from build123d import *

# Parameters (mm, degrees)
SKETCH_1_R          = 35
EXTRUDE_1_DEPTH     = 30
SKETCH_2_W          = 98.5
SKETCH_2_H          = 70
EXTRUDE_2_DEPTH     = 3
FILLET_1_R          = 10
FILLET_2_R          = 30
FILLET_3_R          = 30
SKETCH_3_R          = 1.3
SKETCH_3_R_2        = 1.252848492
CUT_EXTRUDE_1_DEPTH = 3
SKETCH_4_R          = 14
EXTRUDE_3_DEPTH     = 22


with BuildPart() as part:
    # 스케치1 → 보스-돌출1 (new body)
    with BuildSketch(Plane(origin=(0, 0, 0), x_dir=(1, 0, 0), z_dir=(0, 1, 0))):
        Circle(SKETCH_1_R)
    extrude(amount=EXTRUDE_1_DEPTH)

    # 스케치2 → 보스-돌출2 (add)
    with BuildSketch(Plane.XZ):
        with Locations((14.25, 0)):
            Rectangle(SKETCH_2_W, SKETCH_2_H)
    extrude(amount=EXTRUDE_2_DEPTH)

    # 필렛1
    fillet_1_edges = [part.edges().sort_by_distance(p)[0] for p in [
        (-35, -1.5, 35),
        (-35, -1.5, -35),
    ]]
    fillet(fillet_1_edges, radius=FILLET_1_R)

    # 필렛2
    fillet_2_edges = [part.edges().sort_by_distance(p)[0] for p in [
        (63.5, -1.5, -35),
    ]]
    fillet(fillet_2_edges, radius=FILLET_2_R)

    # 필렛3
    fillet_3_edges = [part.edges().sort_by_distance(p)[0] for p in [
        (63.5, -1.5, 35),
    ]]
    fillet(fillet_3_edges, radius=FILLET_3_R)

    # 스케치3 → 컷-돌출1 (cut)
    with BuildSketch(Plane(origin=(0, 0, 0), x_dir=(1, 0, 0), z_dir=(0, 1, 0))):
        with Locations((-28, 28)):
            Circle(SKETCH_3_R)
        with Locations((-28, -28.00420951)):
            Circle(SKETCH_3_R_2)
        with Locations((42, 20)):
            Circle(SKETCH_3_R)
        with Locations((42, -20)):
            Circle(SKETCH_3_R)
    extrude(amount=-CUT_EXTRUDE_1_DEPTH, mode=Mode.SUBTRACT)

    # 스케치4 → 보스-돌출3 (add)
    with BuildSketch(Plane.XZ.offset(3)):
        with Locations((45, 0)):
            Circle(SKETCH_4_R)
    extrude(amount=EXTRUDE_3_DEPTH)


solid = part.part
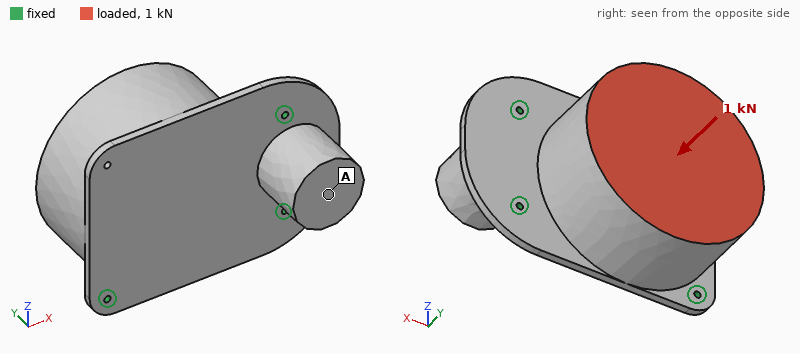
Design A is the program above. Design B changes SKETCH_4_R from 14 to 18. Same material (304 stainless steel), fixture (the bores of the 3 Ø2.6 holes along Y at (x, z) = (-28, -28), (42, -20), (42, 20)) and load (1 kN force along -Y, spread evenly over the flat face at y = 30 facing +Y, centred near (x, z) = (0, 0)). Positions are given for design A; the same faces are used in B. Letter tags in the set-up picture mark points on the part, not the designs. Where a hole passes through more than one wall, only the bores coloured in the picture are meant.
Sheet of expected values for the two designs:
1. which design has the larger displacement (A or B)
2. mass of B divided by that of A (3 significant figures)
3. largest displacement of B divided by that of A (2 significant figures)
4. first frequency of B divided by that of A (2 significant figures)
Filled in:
A
1.06
0.63
1.3
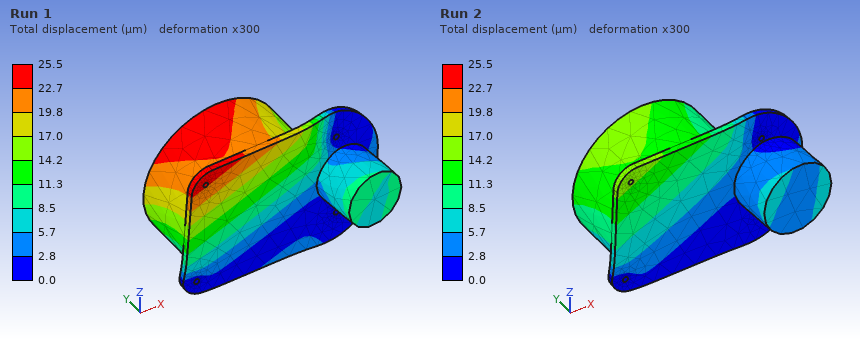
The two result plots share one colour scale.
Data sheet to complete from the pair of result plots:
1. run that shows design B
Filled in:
Run 2
